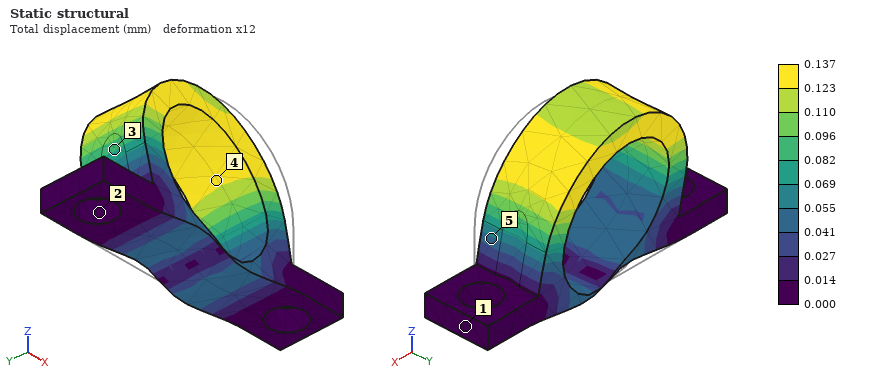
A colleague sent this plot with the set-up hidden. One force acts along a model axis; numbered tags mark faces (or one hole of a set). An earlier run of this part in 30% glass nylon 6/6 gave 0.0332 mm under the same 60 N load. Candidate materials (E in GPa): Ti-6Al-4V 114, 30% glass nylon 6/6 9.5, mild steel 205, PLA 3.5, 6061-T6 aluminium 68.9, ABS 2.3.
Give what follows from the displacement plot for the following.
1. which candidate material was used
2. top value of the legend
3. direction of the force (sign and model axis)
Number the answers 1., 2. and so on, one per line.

1. ABS
2. 0.137 mm
3. -X
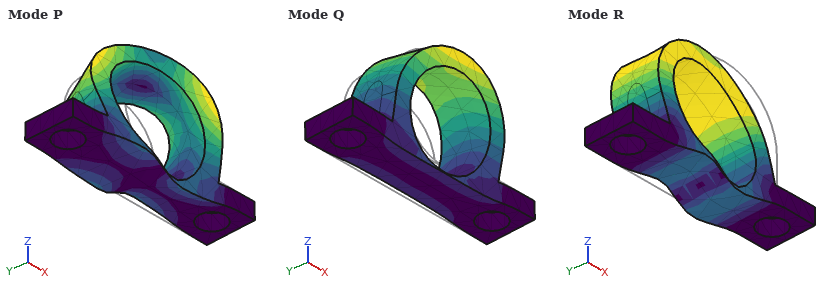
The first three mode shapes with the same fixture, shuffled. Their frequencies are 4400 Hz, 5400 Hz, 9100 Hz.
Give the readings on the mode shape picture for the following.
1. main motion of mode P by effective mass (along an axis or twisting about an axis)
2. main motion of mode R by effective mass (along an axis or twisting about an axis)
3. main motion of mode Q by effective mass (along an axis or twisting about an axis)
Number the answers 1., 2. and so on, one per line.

1. twisting about Z
2. along X
3. along Y
